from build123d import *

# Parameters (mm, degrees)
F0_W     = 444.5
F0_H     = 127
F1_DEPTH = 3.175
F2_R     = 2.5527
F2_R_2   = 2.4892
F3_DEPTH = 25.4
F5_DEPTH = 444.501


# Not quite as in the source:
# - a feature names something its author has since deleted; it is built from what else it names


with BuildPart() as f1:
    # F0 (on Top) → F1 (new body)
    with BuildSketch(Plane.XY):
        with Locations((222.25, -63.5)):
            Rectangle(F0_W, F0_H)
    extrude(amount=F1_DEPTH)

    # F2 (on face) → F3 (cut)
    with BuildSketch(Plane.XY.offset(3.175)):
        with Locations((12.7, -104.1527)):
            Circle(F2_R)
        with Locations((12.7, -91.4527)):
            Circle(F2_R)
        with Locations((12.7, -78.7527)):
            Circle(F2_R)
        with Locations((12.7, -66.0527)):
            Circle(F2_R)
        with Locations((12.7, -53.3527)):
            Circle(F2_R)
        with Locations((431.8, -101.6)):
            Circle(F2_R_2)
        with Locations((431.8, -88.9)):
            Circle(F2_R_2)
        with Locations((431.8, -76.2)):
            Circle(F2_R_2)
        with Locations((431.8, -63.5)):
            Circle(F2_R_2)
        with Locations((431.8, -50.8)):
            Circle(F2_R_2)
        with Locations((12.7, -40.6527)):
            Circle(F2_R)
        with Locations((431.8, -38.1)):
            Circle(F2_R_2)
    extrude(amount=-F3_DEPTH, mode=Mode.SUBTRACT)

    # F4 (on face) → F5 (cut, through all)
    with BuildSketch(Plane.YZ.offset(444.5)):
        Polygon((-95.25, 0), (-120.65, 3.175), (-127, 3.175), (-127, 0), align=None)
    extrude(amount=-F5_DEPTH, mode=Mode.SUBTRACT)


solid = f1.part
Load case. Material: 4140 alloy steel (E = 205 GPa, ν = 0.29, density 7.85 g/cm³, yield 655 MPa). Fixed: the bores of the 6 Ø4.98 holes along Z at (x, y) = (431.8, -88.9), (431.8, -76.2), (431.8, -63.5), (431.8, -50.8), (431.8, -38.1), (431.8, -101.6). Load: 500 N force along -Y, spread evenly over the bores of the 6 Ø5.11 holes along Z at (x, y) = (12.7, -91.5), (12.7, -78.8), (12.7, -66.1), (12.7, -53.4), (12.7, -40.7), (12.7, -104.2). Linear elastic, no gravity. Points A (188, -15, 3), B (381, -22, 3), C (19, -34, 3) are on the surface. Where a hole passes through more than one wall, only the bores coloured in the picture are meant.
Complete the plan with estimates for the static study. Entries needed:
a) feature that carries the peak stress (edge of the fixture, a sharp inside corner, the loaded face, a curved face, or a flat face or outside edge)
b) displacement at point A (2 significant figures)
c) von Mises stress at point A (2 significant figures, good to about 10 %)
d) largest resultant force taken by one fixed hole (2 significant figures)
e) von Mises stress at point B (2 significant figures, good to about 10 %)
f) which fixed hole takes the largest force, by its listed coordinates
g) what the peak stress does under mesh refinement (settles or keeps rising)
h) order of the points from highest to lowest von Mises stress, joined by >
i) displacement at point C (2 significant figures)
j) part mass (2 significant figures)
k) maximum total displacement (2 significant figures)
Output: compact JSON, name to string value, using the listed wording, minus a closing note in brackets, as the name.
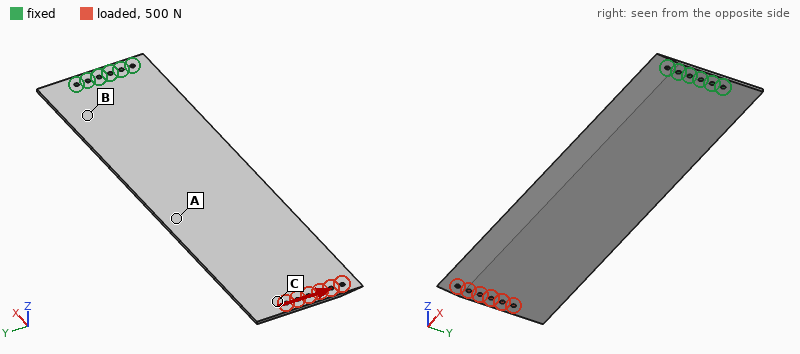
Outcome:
{"feature that carries the peak stress": "edge of the fixture", "displacement at point A": "0.33 mm", "von Mises stress at point A": "12 MPa", "largest resultant force taken by one fixed hole": "3.2 kN", "von Mises stress at point B": "22 MPa", "which fixed hole takes the largest force, by its listed coordinates": "(431.8, -38.1)", "what the peak stress does under mesh refinement": "keeps rising", "order of the points from highest to lowest von Mises stress, joined by >": "B > A > C", "displacement at point C": "0.77 mm", "part mass": "1.2 kg", "maximum total displacement": "0.87 mm"}
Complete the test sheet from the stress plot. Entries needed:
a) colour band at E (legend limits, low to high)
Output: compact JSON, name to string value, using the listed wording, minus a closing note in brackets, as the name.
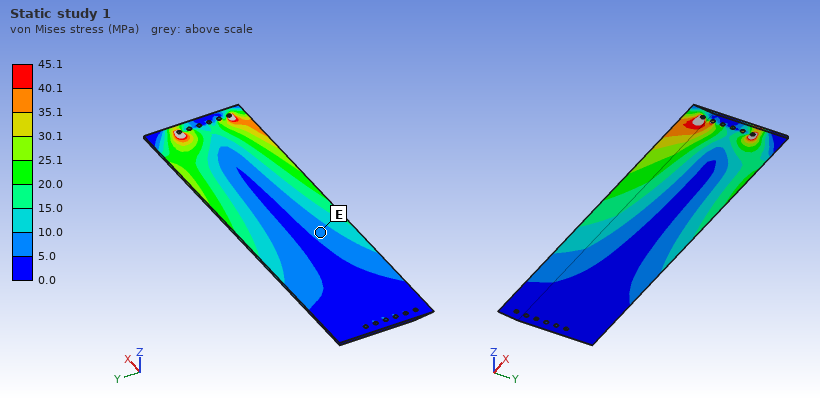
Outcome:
{"colour band at E": "5.0 to 10.0 MPa"}
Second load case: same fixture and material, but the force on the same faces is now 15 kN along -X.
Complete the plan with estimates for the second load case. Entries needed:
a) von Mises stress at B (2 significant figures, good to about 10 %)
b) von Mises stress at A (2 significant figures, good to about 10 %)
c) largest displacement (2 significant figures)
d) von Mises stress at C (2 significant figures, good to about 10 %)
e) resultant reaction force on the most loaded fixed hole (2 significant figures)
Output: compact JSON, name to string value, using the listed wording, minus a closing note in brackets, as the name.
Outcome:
{"von Mises stress at B": "18 MPa", "von Mises stress at A": "11 MPa", "largest displacement": "1.2 mm", "von Mises stress at C": "33 MPa", "resultant reaction force on the most loaded fixed hole": "3.2 kN"}
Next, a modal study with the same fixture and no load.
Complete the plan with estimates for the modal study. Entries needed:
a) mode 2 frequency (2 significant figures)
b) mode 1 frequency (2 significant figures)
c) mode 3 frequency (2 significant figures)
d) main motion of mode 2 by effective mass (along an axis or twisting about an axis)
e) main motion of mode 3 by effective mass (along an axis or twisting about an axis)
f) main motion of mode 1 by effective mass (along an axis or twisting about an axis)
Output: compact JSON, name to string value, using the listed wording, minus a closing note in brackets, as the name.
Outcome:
{"mode 2 frequency": "88 Hz", "mode 1 frequency": "14 Hz", "mode 3 frequency": "110 Hz", "main motion of mode 2 by effective mass": "along Z", "main motion of mode 3 by effective mass": "twisting about X", "main motion of mode 1 by effective mass": "along Z"}
